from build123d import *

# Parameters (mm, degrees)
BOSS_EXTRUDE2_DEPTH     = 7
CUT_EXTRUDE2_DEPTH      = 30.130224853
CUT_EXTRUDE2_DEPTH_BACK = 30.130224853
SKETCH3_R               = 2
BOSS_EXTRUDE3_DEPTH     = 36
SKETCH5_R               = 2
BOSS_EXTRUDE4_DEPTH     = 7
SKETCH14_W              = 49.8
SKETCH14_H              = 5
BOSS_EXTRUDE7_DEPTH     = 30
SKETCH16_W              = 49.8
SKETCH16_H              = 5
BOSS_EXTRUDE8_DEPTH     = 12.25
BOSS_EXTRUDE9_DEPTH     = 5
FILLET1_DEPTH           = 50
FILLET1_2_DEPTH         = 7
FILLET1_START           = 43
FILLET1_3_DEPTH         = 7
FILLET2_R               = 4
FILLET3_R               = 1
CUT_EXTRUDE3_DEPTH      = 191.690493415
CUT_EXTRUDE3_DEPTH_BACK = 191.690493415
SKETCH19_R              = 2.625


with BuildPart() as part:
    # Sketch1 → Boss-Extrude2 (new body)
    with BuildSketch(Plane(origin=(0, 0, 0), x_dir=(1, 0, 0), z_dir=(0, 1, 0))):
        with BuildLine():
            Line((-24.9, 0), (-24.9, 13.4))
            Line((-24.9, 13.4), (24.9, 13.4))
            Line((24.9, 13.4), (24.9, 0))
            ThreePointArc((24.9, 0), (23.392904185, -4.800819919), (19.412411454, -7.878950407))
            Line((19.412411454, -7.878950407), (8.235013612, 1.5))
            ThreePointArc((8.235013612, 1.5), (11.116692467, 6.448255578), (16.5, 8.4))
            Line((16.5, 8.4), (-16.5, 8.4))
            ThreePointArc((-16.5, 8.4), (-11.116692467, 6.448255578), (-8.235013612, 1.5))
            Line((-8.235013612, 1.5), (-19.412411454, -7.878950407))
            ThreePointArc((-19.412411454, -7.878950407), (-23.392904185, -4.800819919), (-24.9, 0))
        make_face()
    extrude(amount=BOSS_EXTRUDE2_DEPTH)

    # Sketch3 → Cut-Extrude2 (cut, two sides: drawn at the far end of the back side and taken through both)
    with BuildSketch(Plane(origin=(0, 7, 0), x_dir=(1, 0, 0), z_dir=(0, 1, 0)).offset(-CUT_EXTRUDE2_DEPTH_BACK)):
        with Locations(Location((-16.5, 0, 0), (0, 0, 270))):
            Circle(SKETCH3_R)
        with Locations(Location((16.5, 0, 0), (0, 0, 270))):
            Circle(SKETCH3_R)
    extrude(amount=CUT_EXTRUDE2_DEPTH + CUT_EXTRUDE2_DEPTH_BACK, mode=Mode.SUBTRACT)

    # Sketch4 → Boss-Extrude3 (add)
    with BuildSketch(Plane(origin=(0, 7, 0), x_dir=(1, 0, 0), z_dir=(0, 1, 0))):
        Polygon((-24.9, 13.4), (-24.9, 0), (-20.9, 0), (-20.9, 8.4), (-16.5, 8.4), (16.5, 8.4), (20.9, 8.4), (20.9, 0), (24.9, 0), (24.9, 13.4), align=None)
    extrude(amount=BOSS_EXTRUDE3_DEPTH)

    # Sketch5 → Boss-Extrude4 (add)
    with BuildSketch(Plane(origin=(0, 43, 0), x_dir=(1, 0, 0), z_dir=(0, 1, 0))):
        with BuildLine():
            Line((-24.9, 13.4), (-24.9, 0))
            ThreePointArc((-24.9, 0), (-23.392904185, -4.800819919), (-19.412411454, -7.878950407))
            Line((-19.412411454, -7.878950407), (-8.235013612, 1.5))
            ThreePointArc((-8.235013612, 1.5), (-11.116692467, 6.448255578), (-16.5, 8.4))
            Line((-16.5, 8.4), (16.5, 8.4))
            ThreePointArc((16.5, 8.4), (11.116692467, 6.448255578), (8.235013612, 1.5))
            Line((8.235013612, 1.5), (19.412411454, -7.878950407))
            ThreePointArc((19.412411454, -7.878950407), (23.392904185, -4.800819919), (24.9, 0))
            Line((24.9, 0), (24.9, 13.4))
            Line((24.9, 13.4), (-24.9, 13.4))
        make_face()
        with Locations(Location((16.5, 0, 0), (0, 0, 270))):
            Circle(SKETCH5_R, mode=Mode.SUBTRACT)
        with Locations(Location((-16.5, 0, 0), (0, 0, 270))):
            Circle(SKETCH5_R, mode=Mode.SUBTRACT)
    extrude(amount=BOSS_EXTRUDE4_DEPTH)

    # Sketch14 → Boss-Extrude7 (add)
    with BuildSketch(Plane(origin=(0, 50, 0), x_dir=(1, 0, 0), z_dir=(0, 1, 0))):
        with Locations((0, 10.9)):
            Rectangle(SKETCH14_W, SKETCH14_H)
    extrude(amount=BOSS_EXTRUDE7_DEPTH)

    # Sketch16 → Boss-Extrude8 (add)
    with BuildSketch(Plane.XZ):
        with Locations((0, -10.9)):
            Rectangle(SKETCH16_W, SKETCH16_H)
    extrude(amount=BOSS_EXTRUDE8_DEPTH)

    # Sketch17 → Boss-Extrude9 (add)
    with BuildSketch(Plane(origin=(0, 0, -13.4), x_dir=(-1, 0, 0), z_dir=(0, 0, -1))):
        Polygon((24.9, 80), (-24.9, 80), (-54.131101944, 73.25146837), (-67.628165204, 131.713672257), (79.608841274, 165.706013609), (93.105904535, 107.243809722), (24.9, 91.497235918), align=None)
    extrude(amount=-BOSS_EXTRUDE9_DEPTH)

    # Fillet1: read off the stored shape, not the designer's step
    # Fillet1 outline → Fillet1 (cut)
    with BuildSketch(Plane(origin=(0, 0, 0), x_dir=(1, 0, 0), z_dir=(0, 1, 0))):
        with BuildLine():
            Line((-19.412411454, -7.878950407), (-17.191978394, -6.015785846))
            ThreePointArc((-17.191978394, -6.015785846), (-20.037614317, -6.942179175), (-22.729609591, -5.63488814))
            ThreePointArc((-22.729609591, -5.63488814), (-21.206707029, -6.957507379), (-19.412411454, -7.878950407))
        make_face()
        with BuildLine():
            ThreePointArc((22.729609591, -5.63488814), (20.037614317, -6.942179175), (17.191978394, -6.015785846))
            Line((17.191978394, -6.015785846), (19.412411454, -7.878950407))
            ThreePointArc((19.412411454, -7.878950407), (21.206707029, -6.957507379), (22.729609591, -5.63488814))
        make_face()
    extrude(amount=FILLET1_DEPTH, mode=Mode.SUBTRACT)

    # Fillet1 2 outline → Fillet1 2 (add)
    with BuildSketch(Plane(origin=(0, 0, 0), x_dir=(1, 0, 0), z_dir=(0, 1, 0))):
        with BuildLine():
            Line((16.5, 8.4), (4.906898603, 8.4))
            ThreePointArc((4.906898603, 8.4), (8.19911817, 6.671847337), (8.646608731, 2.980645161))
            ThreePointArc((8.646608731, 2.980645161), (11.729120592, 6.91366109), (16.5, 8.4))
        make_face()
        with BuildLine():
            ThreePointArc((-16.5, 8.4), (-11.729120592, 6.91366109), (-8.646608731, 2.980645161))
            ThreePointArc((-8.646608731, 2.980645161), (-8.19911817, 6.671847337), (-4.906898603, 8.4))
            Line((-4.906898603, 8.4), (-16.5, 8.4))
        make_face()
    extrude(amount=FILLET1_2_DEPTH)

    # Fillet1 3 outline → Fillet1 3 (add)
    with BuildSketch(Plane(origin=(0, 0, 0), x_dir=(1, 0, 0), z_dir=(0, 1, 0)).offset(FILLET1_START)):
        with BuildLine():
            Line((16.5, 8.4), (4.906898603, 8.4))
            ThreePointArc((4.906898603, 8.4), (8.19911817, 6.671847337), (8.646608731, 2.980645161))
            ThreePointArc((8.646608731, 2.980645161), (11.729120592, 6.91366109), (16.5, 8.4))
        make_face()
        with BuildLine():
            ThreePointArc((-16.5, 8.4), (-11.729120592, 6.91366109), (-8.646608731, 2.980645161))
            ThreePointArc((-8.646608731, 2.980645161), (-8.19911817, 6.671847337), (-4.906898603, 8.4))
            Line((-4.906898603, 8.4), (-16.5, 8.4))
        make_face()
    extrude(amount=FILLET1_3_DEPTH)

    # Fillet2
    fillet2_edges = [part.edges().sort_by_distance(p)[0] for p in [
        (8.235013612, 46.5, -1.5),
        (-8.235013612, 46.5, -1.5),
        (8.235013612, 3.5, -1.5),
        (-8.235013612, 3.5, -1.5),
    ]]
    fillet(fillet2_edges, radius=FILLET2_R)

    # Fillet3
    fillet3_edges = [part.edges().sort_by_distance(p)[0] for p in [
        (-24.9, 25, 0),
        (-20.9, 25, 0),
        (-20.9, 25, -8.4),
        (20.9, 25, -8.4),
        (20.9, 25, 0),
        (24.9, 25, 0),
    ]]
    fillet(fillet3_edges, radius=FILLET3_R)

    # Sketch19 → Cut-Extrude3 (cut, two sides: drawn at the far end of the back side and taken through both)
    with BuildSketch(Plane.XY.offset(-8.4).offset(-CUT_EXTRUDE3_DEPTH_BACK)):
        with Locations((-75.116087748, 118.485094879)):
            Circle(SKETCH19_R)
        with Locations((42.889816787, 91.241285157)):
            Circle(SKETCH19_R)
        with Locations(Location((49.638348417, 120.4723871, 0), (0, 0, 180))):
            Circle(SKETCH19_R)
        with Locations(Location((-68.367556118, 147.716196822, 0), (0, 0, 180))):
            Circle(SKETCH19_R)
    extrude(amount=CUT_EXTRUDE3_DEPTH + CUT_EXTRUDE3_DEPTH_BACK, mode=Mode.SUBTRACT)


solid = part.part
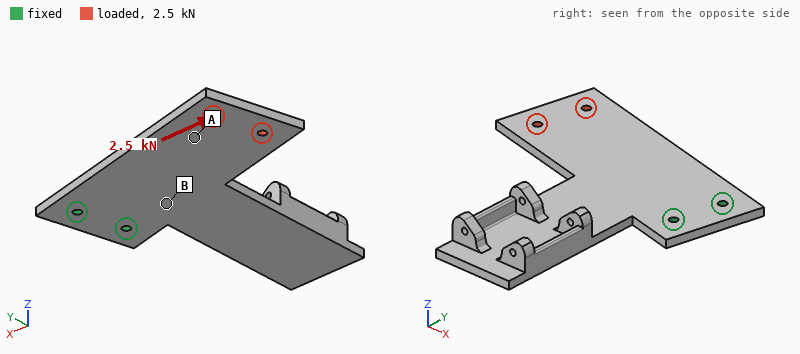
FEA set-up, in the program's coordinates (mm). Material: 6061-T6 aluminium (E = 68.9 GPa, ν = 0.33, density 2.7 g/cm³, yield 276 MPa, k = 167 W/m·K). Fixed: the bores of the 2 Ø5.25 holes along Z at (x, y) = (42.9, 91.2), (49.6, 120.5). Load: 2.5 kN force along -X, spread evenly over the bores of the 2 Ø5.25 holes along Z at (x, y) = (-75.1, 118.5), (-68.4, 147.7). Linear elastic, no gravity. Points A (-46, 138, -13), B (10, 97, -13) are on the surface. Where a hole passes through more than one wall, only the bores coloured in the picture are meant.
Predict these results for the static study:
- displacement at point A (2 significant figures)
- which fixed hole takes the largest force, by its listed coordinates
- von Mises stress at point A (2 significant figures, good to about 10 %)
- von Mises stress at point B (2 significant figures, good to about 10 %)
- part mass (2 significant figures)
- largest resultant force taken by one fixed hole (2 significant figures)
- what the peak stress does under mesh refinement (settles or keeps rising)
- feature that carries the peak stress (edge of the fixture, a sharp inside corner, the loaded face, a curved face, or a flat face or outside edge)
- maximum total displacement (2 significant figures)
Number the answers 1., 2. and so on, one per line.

1. 63 µm
2. (49.6, 120.5)
3. 11 MPa
4. 4.4 MPa
5. 210 g
6. 3.3 kN
7. keeps rising
8. edge of the fixture
9. 98 µm
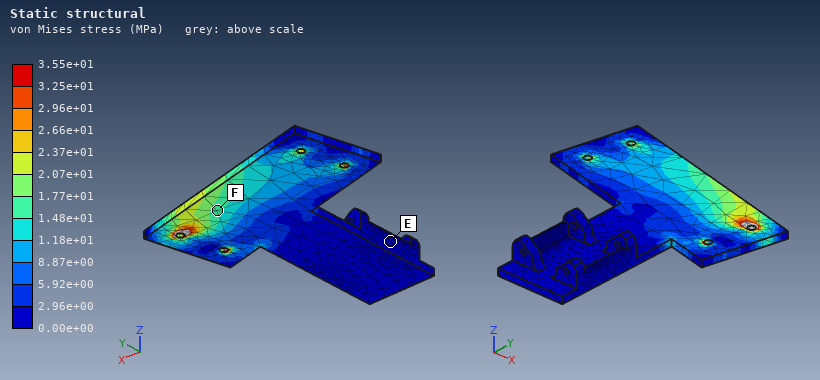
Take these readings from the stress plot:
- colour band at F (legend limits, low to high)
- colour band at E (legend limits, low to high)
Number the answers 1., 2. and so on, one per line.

1. 1.48e+01 to 1.77e+01 MPa
2. 0.00e+00 to 2.96e+00 MPa
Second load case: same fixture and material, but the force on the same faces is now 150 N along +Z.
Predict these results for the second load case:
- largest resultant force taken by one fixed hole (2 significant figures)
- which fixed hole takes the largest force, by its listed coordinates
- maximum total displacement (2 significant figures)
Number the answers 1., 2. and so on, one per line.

1. 83 N
2. (42.9, 91.2)
3. 2.2 mm
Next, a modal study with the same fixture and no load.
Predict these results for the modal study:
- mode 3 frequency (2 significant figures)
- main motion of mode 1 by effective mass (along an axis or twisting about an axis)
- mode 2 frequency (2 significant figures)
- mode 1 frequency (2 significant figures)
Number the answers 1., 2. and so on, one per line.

1. 890 Hz
2. along Z
3. 240 Hz
4. 230 Hz
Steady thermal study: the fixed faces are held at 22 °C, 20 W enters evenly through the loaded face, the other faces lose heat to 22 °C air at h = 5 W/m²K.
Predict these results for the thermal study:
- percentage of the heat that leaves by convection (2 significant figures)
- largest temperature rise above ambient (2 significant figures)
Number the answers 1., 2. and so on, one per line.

1. 15 %
2. 45 K
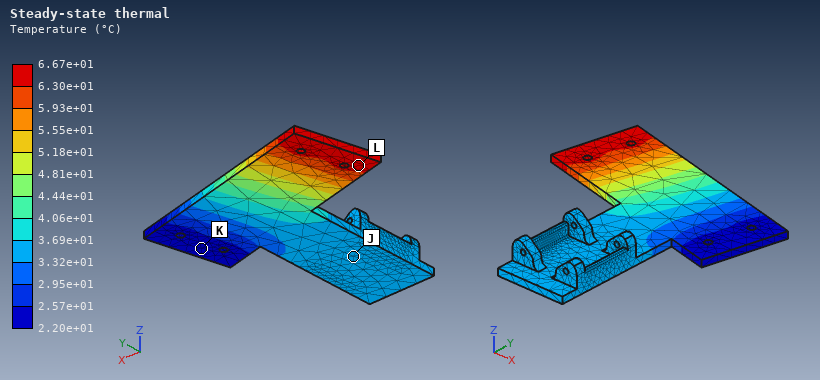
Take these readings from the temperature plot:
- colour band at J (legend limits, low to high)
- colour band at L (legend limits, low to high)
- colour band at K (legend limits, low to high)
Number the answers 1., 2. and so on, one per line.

1. 3.32e+01 to 3.69e+01 °C
2. 6.30e+01 to 6.67e+01 °C
3. 2.20e+01 to 2.57e+01 °C
